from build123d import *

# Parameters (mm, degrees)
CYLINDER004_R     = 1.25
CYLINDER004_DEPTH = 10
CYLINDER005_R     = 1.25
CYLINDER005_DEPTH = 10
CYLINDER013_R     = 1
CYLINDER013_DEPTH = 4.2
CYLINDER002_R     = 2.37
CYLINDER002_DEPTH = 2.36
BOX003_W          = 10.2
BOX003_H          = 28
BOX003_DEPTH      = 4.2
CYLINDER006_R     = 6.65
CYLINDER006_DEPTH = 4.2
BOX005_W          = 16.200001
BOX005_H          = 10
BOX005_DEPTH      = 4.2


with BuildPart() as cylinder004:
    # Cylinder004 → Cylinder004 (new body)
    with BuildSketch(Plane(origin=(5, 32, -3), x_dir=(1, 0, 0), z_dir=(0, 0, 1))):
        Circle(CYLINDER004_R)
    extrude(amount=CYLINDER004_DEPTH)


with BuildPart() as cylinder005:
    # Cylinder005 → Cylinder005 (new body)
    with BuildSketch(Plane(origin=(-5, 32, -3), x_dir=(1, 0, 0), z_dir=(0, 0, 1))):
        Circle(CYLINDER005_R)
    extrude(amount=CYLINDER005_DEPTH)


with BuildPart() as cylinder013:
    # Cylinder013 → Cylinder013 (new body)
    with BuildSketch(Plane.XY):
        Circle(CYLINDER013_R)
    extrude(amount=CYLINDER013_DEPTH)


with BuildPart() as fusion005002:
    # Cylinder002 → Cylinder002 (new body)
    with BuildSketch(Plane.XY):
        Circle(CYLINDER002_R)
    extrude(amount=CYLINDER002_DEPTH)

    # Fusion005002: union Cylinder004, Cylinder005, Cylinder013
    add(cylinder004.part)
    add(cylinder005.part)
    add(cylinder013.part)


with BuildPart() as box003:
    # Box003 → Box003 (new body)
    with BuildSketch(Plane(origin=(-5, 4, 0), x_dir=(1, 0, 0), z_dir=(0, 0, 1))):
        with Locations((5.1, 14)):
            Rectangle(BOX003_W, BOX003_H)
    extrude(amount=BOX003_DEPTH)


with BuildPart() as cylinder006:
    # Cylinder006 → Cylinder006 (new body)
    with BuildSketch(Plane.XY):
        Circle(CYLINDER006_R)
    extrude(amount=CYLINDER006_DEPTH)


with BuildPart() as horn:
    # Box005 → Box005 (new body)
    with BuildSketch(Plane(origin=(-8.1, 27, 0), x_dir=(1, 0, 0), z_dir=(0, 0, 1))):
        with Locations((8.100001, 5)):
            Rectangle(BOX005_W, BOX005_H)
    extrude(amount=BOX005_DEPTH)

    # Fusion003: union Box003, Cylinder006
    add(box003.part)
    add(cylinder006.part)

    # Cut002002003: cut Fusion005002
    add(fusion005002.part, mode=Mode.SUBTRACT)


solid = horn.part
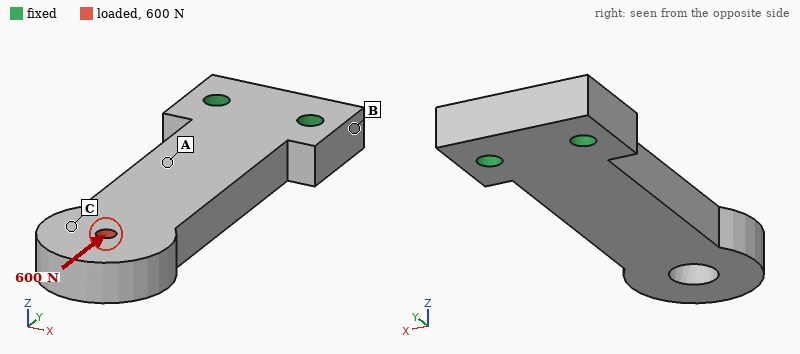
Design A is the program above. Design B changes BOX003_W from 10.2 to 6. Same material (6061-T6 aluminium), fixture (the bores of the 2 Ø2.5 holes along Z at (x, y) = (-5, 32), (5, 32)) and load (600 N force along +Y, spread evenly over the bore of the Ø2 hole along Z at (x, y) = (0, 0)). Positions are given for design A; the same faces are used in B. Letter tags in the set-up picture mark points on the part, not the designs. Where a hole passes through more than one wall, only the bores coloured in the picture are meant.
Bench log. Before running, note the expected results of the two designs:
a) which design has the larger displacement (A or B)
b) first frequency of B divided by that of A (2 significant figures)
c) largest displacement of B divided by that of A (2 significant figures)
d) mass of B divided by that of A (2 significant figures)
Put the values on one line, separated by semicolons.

B; 0.82; 1.6; 0.82
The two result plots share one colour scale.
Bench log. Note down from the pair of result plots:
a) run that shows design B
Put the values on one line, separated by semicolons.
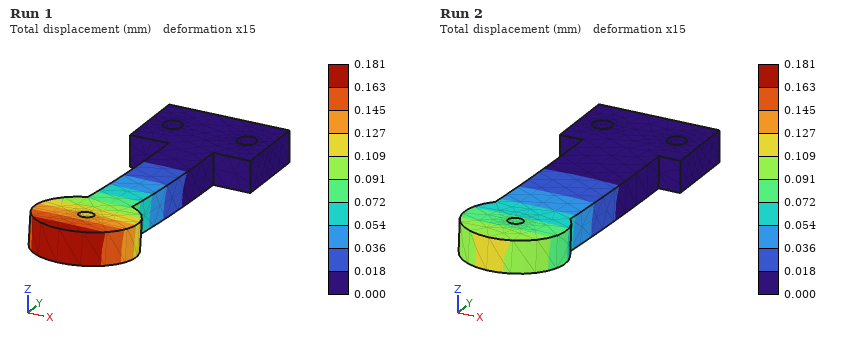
Run 1
